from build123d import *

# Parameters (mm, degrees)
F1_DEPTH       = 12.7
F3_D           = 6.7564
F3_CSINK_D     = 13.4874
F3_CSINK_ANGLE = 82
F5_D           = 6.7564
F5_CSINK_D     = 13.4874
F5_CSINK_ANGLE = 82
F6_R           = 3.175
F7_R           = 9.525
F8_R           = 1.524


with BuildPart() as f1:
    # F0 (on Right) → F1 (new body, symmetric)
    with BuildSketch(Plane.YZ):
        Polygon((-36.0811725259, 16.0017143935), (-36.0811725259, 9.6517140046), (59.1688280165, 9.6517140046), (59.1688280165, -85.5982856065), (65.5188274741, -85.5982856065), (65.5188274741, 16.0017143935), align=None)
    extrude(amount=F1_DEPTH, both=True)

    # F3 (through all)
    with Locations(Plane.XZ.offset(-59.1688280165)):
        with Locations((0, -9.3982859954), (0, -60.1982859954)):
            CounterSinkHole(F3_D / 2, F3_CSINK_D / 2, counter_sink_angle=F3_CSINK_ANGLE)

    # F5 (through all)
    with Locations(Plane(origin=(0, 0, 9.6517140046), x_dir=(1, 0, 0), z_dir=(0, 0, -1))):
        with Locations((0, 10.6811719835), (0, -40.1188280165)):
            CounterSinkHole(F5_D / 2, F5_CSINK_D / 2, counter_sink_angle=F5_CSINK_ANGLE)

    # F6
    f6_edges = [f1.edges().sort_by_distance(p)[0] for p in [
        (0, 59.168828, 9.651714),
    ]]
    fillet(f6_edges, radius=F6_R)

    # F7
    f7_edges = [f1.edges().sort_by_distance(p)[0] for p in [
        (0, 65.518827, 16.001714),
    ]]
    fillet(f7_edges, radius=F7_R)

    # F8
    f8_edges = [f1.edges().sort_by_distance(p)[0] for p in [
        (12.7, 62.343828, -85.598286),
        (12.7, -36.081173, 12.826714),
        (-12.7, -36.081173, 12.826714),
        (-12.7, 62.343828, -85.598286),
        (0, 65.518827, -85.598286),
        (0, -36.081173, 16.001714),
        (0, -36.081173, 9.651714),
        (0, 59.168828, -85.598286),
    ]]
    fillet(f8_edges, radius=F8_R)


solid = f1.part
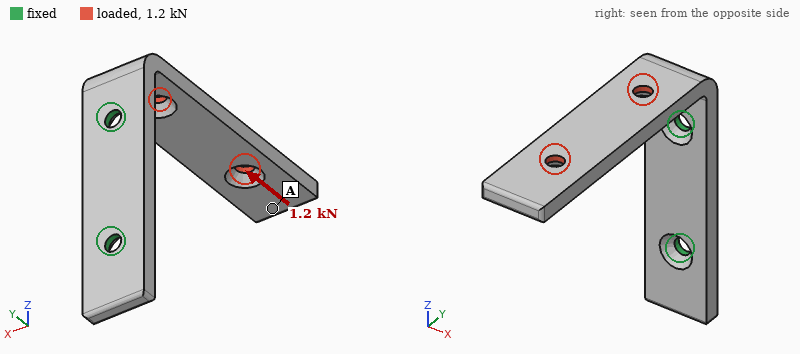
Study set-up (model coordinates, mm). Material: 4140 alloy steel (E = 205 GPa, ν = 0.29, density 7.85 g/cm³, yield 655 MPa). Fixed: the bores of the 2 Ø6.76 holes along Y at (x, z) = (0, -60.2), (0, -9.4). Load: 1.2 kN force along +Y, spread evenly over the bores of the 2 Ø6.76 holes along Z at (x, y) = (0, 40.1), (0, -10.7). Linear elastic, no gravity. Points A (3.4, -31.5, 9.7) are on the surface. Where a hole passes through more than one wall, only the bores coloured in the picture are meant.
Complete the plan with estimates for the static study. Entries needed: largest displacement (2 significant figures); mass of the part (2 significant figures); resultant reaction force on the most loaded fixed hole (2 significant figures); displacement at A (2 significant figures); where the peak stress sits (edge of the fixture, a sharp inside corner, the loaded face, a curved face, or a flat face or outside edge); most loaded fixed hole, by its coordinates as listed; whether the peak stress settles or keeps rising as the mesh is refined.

0.52 mm
230 g
1.8 kN
0.49 mm
edge of the fixture
(0, -9.4)
keeps rising
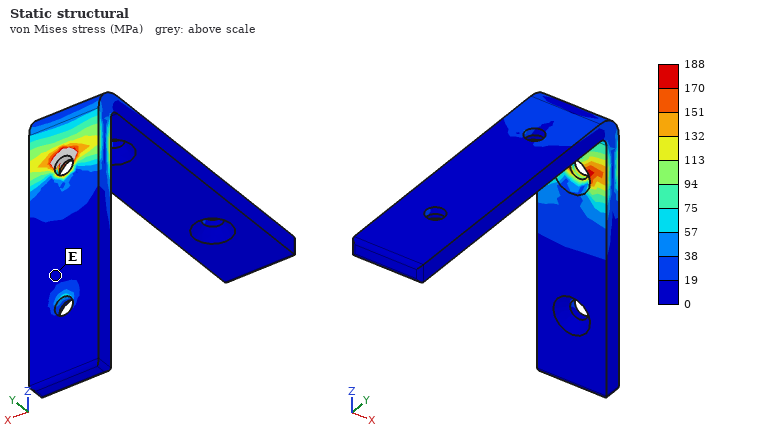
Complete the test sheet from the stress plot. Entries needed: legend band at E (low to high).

0 to 19 MPa
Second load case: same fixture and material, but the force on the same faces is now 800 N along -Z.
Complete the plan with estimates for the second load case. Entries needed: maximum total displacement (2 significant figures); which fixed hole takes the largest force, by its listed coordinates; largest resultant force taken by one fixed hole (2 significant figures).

1.7 mm
(0, -60.2)
1.8 kN
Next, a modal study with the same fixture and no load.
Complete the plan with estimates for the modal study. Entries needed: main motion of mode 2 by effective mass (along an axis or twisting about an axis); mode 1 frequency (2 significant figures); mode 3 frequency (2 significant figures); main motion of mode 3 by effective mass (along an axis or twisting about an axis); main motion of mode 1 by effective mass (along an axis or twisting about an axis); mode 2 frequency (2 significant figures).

along X
370 Hz
2100 Hz
along Y
along Z
570 Hz
